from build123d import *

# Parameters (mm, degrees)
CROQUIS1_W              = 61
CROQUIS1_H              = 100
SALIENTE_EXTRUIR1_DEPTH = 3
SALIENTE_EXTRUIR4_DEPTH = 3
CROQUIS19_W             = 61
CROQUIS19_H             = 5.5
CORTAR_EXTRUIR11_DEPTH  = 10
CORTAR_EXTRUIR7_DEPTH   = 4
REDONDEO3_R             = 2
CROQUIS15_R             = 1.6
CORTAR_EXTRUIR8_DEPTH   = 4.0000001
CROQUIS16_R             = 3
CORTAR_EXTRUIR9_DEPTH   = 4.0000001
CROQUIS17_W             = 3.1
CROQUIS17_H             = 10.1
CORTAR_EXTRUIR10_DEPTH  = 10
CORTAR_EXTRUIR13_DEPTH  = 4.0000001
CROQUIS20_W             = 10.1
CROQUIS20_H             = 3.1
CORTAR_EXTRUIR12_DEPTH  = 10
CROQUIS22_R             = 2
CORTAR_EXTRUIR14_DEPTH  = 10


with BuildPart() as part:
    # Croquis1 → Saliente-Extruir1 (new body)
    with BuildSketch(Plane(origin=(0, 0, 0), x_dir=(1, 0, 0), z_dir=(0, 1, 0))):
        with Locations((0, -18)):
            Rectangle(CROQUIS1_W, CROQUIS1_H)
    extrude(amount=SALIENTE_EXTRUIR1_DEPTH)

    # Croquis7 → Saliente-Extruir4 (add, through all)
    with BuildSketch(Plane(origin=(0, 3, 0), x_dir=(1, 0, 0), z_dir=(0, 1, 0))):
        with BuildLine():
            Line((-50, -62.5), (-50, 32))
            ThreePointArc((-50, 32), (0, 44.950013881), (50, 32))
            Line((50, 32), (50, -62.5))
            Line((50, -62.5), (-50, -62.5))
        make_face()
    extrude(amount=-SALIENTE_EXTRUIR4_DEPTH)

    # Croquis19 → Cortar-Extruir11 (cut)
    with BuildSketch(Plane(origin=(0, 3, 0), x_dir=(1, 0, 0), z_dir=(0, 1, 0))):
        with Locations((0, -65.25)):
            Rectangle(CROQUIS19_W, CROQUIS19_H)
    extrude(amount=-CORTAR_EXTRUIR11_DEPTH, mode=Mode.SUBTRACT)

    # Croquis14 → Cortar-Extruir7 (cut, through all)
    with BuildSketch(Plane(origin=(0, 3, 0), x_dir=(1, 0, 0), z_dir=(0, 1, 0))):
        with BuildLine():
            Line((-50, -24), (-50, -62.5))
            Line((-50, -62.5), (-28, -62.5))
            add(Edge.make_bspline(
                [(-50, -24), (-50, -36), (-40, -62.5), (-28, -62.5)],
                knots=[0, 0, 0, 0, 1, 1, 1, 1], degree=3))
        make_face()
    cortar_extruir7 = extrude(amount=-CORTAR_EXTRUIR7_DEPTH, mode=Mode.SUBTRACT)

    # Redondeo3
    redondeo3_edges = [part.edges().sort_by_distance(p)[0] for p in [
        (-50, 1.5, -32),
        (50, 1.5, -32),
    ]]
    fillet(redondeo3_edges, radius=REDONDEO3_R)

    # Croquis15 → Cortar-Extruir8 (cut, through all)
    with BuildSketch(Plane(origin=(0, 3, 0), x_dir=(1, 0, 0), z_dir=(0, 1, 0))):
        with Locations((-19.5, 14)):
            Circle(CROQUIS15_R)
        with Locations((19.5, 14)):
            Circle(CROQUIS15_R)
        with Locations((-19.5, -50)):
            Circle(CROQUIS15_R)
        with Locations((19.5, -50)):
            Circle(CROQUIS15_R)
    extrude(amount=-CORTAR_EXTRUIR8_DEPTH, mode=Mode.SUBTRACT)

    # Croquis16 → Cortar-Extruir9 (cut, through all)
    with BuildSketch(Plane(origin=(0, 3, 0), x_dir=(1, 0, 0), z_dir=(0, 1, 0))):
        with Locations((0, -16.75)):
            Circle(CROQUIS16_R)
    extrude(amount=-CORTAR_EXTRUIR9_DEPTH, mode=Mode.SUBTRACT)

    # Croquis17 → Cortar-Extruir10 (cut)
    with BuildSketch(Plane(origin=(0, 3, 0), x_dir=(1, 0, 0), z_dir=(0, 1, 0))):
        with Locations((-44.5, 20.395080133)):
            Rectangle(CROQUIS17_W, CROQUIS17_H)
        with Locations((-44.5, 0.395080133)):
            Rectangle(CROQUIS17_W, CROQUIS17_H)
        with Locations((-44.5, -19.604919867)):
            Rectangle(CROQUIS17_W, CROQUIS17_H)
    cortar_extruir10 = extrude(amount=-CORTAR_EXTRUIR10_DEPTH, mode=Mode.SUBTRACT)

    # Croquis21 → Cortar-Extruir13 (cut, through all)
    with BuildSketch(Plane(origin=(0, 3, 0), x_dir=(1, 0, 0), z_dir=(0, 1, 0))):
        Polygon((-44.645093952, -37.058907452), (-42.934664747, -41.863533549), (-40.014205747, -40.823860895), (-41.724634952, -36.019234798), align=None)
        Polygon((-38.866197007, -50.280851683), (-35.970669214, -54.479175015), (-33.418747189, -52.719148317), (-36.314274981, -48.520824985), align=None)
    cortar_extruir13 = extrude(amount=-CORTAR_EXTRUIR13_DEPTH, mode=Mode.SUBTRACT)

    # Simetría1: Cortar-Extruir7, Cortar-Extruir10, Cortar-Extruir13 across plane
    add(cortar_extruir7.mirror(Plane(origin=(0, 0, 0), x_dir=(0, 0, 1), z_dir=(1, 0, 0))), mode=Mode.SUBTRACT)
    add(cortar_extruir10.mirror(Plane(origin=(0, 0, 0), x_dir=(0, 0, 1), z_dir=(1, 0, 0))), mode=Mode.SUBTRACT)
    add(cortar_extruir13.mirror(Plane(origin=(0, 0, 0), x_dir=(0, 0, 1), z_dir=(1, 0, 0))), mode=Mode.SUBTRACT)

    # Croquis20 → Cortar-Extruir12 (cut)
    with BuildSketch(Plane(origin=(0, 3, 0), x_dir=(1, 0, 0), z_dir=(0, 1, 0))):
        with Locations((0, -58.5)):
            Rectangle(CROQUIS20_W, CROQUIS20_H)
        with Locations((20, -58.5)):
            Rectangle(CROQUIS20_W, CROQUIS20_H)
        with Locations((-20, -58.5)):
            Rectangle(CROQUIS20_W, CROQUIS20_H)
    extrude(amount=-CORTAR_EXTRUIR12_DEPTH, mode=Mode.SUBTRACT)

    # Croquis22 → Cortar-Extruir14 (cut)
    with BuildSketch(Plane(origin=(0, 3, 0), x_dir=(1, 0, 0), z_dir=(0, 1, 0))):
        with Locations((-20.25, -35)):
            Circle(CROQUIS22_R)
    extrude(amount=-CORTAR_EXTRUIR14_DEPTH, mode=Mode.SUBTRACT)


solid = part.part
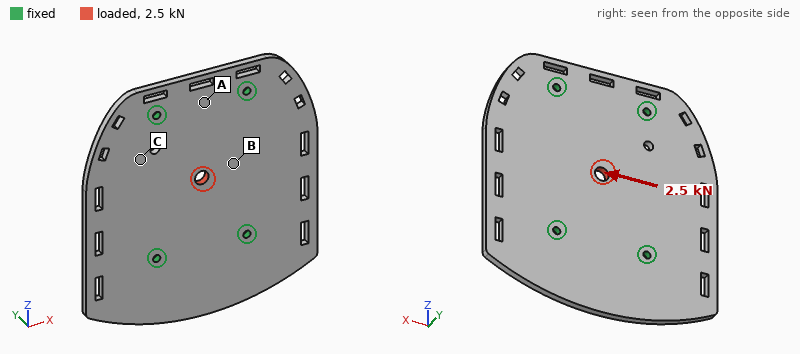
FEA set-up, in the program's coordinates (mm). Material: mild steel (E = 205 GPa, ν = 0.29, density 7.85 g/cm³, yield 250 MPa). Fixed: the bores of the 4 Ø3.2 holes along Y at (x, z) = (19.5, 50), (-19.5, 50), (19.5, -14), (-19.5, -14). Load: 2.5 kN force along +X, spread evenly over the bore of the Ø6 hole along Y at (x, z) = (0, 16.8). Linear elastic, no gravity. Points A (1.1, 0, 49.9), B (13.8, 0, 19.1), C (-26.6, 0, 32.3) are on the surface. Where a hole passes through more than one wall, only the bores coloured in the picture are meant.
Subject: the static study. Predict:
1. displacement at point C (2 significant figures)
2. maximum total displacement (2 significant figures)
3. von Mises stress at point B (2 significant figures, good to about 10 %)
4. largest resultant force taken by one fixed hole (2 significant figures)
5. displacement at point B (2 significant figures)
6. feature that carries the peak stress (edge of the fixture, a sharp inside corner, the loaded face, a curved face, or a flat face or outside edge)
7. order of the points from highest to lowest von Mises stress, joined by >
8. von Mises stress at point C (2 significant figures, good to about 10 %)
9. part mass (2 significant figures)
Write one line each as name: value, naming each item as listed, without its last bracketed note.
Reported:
displacement at point C: 1.6 µm
maximum total displacement: 4.0 µm
von Mises stress at point B: 15 MPa
largest resultant force taken by one fixed hole: 680 N
displacement at point B: 2.6 µm
feature that carries the peak stress: the loaded face
order of the points from highest to lowest von Mises stress, joined by >: B > C > A
von Mises stress at point C: 7.7 MPa
part mass: 220 g
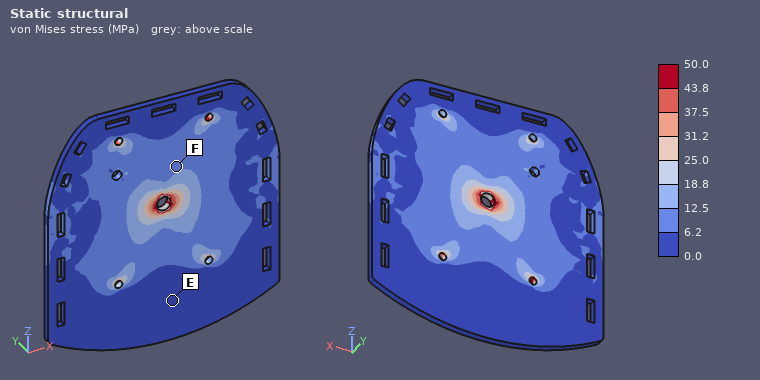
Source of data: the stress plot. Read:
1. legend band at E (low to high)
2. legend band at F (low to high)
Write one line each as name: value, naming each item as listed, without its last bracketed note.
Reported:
legend band at E: 0.0 to 6.2 MPa
legend band at F: 6.2 to 12.5 MPa
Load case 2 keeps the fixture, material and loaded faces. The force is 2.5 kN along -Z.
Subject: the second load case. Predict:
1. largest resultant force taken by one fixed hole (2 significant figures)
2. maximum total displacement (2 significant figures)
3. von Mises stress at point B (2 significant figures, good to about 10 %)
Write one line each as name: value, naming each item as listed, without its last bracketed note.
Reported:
largest resultant force taken by one fixed hole: 690 N
maximum total displacement: 3.3 µm
von Mises stress at point B: 6.0 MPa
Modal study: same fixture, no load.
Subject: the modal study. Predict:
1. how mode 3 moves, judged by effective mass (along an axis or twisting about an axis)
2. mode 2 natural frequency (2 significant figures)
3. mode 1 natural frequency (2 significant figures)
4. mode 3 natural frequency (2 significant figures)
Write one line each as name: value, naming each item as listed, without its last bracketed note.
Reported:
how mode 3 moves, judged by effective mass: along Y
mode 2 natural frequency: 2200 Hz
mode 1 natural frequency: 2100 Hz
mode 3 natural frequency: 2500 Hz
